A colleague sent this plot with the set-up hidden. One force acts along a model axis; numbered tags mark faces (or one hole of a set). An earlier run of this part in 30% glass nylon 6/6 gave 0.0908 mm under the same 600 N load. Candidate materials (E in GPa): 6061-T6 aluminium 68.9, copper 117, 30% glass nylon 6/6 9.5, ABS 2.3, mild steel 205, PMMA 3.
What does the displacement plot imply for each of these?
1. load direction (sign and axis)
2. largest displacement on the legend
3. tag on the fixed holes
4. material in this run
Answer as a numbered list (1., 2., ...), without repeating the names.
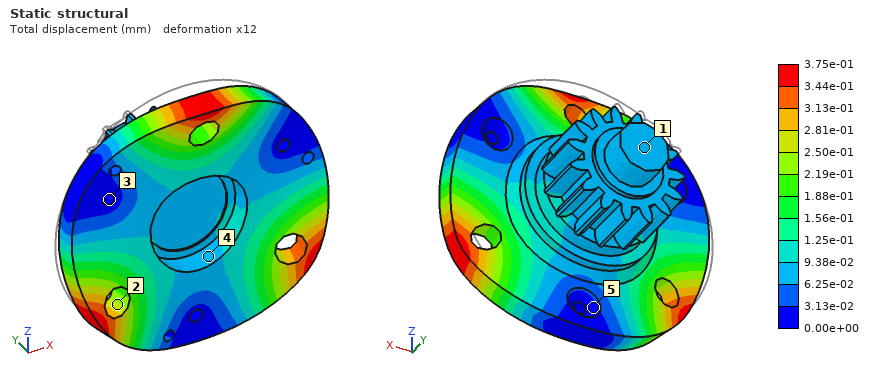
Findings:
1. -Y
2. 3.75e-01 mm
3. 3
4. ABS
